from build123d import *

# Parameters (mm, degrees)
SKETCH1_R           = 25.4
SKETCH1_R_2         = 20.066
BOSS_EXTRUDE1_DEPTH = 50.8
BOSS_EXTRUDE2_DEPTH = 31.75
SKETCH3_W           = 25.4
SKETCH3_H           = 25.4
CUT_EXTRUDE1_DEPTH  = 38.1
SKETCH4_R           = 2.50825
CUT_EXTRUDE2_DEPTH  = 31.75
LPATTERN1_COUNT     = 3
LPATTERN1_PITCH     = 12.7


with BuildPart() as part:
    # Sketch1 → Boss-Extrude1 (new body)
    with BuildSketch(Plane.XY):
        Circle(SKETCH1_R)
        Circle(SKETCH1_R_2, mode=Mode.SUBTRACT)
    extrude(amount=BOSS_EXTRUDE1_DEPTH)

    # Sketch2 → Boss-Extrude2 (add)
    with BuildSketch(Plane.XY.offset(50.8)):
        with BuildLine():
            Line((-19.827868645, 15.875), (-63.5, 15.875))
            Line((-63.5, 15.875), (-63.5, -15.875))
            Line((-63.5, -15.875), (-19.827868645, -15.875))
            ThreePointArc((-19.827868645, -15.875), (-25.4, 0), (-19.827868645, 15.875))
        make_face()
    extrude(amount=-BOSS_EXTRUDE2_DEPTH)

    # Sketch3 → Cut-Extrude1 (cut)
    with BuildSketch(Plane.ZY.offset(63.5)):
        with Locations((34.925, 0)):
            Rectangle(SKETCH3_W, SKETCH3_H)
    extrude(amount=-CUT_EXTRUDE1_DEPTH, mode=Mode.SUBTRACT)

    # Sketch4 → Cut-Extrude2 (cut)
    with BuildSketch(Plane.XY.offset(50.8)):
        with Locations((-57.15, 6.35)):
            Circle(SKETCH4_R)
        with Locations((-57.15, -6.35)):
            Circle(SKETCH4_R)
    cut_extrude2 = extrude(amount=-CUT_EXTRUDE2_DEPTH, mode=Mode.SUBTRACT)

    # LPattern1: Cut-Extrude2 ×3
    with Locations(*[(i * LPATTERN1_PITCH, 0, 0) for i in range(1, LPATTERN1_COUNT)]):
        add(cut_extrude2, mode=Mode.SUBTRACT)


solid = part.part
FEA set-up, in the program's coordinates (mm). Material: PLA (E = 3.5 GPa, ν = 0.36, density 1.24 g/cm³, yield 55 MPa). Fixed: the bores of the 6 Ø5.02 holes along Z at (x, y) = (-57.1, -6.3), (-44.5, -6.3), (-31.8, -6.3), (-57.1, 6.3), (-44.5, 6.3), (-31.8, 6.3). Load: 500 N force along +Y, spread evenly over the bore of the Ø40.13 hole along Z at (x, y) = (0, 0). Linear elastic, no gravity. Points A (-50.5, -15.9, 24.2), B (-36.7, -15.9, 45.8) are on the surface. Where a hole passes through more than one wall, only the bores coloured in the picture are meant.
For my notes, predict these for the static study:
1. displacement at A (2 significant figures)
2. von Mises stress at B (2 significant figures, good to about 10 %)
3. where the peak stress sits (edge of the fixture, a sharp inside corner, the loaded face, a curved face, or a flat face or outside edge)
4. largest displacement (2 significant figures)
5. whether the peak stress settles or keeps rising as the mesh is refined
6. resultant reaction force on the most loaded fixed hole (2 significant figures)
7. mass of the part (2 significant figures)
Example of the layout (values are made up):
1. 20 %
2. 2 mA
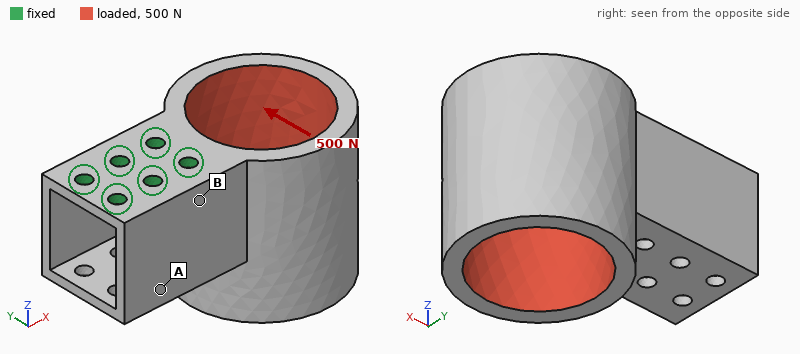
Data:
1. 0.29 mm
2. 6.9 MPa
3. edge of the fixture
4. 1.2 mm
5. keeps rising
6. 600 N
7. 66 g
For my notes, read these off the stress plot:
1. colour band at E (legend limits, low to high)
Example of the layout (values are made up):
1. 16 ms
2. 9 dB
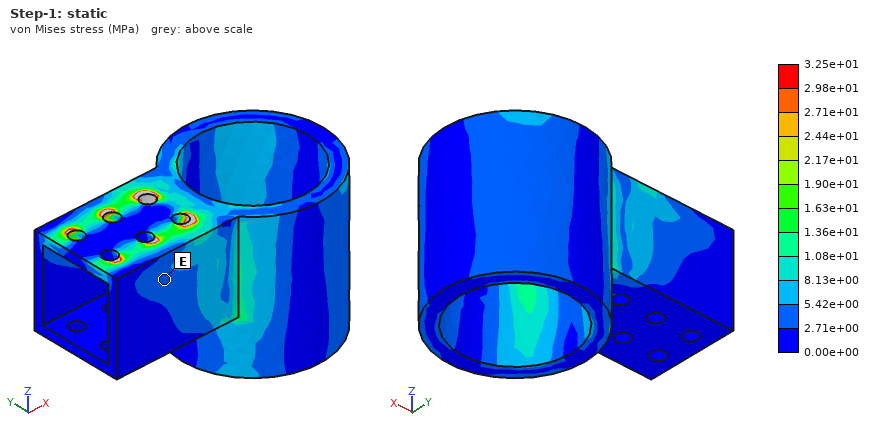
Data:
1. 2.71e+00 to 5.42e+00 MPa
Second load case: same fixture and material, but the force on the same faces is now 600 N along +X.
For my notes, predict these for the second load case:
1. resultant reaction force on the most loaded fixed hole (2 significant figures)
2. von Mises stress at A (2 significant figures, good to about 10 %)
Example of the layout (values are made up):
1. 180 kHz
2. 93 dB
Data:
1. 280 N
2. 4.0 MPa
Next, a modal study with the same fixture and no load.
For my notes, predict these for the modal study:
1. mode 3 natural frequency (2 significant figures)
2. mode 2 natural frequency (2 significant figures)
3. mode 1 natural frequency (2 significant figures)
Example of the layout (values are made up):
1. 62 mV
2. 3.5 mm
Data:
1. 690 Hz
2. 560 Hz
3. 550 Hz
